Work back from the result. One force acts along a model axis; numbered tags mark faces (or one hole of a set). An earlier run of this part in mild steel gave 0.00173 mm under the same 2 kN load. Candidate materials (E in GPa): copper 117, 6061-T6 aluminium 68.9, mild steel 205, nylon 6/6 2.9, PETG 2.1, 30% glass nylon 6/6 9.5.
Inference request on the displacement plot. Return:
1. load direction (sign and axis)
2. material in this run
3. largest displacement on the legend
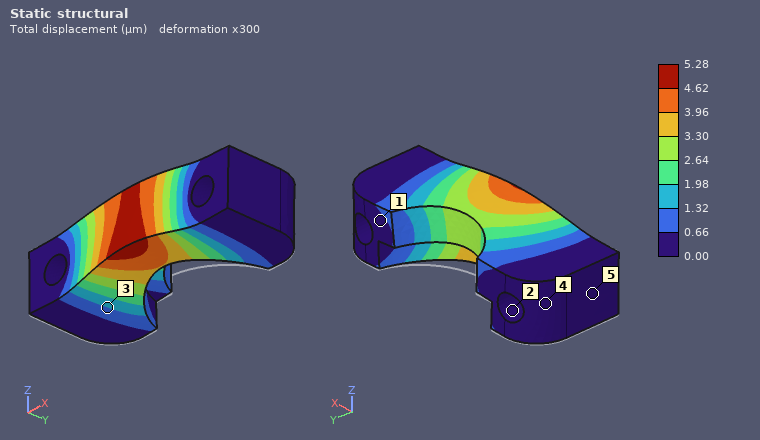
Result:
+Z
6061-T6 aluminium
5.28 µm
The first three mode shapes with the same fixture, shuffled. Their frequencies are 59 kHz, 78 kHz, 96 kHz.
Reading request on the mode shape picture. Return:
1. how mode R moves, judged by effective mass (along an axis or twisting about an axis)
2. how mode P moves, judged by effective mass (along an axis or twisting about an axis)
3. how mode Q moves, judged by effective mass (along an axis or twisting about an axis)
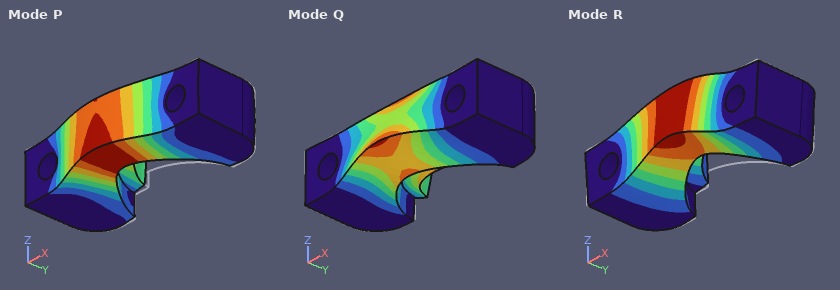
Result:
along Z
along Y
twisting about X
